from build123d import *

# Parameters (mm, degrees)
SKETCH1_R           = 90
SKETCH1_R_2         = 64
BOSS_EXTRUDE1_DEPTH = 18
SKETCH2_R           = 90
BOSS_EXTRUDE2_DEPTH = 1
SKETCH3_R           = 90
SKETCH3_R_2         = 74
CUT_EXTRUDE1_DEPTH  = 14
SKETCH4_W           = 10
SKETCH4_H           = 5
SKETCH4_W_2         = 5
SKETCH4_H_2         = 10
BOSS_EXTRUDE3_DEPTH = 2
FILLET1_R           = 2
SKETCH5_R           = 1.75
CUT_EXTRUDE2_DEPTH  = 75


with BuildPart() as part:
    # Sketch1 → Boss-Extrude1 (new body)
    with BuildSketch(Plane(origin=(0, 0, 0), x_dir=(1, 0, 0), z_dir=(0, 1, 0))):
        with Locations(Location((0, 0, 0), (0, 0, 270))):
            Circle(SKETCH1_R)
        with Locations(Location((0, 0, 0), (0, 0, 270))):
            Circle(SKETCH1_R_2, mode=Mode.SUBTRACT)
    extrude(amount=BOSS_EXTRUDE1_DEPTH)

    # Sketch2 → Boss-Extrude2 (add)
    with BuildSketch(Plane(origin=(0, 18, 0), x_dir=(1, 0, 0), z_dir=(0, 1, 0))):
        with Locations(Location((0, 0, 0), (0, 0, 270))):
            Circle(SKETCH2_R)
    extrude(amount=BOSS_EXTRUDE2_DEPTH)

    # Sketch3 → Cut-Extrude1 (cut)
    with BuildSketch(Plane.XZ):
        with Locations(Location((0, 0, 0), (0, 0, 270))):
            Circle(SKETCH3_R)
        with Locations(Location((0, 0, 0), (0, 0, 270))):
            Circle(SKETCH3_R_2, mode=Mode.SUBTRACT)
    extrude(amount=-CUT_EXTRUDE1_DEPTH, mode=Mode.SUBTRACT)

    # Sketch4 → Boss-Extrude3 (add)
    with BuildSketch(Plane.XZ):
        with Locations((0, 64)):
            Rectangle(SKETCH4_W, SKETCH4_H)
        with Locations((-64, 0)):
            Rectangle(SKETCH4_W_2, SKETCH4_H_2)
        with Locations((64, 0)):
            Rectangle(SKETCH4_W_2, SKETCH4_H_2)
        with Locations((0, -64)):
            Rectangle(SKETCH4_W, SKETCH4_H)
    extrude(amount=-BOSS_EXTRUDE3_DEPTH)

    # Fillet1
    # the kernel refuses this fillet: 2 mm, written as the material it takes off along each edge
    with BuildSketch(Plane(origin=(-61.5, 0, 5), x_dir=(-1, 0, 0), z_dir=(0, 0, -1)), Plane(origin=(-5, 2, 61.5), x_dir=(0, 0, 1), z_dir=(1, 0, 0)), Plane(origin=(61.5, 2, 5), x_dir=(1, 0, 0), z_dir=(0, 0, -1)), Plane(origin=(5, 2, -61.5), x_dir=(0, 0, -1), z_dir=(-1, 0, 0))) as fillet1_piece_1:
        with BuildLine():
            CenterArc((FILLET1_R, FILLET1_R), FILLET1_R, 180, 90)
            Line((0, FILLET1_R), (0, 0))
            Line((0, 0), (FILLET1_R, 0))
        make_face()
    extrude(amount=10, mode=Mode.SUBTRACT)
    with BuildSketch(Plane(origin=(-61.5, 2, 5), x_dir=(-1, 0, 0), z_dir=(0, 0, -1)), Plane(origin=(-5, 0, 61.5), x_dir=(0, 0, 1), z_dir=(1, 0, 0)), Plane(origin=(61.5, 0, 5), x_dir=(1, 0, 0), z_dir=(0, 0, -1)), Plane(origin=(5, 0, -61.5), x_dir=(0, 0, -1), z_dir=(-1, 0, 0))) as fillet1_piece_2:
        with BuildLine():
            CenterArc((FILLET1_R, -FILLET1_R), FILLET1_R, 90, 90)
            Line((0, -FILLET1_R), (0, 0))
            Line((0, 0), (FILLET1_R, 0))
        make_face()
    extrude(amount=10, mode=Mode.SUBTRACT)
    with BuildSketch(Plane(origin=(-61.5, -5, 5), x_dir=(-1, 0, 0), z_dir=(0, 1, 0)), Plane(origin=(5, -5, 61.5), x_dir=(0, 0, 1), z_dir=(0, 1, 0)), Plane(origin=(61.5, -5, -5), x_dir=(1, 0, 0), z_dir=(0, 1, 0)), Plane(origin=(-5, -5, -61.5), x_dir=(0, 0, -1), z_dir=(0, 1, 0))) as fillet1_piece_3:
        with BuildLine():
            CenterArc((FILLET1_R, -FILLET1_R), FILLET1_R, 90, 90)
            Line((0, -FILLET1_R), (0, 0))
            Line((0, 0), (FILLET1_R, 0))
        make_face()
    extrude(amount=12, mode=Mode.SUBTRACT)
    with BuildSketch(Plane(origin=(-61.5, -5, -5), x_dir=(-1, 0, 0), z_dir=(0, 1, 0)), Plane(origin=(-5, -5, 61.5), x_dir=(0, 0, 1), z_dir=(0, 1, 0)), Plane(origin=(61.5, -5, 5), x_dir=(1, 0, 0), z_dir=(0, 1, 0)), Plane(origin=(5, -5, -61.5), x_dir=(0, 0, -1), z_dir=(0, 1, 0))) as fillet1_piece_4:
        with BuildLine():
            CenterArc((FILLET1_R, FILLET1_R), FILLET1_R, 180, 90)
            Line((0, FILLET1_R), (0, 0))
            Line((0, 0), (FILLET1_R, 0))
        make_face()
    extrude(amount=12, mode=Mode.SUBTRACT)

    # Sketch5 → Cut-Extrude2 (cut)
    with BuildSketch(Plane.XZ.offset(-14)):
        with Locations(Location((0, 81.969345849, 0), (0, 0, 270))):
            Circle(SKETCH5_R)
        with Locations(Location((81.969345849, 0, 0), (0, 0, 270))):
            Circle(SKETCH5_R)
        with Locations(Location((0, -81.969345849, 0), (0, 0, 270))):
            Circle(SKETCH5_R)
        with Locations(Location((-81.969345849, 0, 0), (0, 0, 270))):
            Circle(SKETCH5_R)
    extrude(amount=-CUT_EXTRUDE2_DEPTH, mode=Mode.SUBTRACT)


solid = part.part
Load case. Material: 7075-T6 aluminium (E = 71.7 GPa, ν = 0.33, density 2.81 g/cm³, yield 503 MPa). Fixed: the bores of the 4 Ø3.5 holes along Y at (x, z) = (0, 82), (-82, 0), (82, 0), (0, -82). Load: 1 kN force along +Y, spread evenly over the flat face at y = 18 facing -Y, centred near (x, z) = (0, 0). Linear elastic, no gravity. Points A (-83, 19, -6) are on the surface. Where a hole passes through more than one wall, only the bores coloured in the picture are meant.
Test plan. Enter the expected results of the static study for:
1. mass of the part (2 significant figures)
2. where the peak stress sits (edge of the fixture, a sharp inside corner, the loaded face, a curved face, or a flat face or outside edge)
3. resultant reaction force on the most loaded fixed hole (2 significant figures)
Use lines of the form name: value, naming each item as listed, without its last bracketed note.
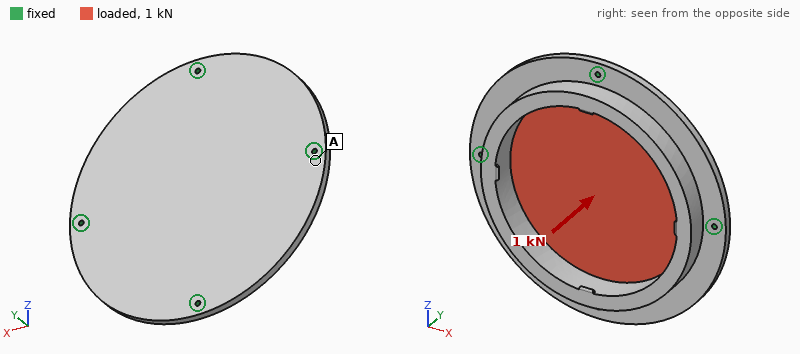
mass of the part: 380 g
where the peak stress sits: a flat face or outside edge
resultant reaction force on the most loaded fixed hole: 300 N
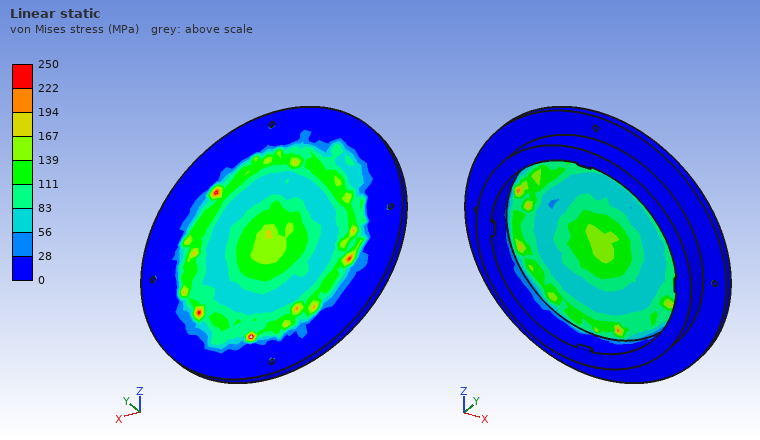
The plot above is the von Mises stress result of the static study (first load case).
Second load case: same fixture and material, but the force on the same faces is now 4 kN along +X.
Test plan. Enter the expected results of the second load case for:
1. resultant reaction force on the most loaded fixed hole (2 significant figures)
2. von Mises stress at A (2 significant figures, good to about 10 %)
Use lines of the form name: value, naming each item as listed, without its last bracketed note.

resultant reaction force on the most loaded fixed hole: 1.0 kN
von Mises stress at A: 7.5 MPa
